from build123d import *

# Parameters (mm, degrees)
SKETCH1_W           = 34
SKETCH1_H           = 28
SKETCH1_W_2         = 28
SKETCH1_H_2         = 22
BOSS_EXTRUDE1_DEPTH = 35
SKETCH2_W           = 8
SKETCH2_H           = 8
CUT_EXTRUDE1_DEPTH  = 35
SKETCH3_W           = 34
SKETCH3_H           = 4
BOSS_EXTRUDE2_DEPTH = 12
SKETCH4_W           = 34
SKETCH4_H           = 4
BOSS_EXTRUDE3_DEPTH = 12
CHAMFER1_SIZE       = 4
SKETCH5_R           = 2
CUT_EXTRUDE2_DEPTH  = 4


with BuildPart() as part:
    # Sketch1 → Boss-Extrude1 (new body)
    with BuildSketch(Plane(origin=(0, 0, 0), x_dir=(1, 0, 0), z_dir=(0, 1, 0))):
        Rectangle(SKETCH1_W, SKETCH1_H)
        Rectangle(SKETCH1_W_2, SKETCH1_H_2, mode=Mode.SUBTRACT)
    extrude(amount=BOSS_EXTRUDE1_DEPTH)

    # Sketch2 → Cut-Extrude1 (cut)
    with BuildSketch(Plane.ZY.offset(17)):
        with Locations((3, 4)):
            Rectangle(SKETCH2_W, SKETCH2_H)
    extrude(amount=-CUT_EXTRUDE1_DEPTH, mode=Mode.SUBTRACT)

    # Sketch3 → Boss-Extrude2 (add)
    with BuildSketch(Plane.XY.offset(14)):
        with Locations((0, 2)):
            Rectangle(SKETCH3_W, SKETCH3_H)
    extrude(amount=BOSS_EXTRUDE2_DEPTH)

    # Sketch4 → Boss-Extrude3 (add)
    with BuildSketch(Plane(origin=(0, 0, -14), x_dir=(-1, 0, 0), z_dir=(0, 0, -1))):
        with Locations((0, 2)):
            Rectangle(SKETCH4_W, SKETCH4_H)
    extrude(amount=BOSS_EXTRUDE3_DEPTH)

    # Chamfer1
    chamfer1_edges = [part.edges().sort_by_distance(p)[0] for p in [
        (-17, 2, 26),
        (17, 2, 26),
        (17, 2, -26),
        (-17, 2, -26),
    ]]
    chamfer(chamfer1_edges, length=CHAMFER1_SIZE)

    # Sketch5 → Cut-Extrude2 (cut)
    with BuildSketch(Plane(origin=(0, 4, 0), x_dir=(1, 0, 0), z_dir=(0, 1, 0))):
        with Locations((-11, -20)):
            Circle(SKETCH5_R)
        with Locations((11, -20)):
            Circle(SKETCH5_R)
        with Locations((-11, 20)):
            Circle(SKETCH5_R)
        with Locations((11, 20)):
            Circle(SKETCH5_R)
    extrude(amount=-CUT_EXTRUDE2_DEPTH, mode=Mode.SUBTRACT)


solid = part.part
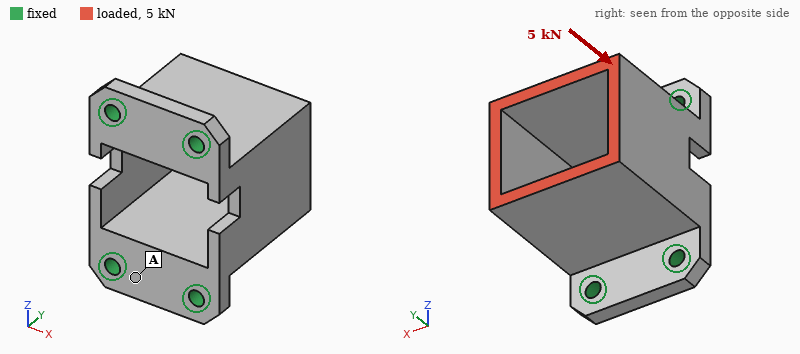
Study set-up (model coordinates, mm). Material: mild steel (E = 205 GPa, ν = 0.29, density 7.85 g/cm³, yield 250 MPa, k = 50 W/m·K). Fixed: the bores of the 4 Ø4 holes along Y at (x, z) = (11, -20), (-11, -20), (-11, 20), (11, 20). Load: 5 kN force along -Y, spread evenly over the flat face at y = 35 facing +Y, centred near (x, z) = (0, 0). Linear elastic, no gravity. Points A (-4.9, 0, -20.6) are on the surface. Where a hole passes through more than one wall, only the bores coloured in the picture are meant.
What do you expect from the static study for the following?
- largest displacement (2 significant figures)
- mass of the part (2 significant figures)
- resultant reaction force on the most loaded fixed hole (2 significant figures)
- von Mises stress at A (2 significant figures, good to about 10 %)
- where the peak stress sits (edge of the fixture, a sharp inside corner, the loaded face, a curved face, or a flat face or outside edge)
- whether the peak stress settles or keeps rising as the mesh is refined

9.8 µm
110 g
1.3 kN
30 MPa
edge of the fixture
keeps rising
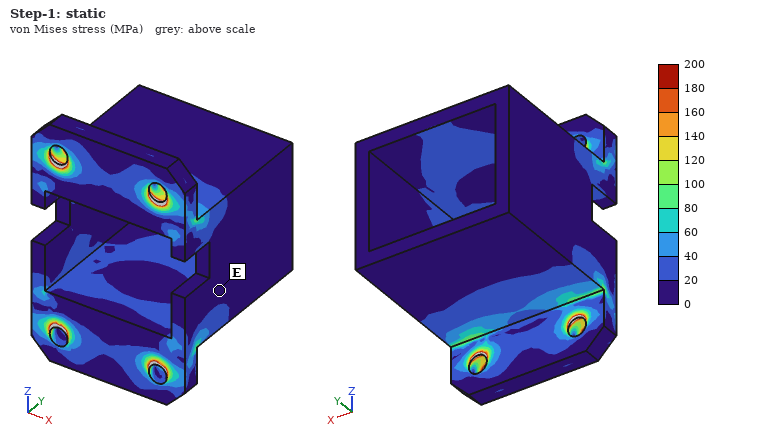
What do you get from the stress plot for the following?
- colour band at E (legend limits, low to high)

0 to 20 MPa
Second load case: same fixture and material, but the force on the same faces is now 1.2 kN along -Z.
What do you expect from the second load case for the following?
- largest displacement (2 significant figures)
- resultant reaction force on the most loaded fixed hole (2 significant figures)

24 µm
700 N
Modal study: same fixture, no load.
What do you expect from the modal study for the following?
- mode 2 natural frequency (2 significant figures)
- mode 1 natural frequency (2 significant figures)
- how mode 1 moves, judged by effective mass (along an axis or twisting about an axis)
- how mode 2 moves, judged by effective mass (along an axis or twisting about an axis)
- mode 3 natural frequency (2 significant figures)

8400 Hz
6600 Hz
along X
along Z
9100 Hz
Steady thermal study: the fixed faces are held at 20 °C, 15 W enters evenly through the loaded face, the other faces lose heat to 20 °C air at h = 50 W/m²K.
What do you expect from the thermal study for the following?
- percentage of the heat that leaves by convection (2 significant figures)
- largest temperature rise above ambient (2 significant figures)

42 %
29 K
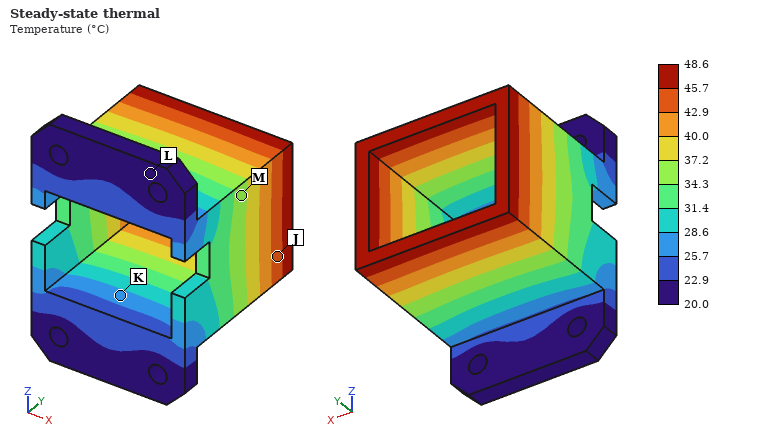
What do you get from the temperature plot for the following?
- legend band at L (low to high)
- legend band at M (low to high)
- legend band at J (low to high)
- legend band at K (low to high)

20.0 to 22.9 °C
34.3 to 37.2 °C
42.9 to 45.7 °C
25.7 to 28.6 °C
